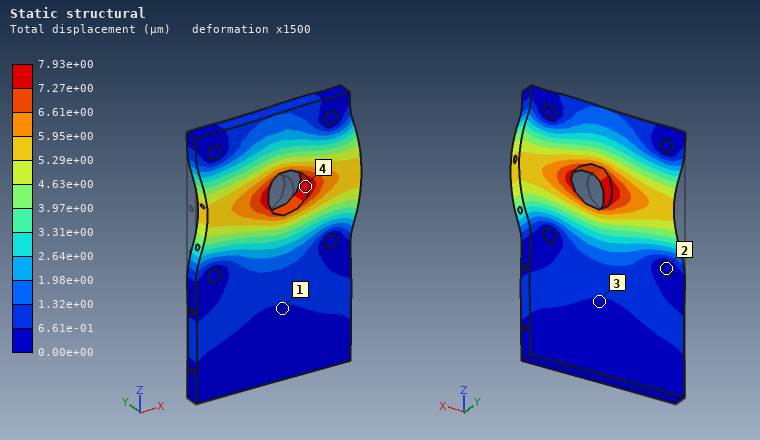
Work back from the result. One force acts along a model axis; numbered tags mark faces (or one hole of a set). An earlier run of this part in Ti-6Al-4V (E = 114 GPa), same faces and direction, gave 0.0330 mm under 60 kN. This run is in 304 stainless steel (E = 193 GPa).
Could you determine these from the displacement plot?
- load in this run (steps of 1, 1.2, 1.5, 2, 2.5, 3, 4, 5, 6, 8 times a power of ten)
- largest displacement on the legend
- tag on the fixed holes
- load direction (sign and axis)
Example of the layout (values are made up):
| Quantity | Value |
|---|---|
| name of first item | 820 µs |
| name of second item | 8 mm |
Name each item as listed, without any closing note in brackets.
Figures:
| Quantity | Value |
|---|---|
| load in this run | 25 kN |
| largest displacement on the legend | 7.93e+00 µm |
| tag on the fixed holes | 2 |
| load direction | +X |
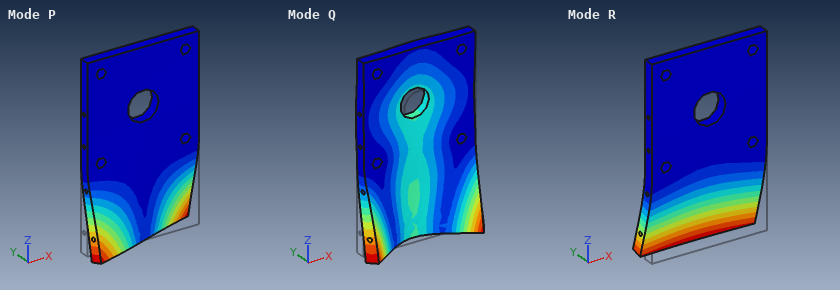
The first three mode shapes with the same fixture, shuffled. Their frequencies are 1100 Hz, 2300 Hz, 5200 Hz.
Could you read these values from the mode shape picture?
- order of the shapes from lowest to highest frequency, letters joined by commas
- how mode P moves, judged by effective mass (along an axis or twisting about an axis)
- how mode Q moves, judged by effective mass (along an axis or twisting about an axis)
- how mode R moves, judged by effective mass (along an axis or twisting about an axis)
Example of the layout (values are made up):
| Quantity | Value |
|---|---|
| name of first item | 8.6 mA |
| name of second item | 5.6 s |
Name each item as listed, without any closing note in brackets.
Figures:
| Quantity | Value |
|---|---|
| order of the shapes from lowest to highest frequency, letters joined by commas | R, P, Q |
| how mode P moves, judged by effective mass | twisting about Z |
| how mode Q moves, judged by effective mass | along Y |
| how mode R moves, judged by effective mass | along Y |
